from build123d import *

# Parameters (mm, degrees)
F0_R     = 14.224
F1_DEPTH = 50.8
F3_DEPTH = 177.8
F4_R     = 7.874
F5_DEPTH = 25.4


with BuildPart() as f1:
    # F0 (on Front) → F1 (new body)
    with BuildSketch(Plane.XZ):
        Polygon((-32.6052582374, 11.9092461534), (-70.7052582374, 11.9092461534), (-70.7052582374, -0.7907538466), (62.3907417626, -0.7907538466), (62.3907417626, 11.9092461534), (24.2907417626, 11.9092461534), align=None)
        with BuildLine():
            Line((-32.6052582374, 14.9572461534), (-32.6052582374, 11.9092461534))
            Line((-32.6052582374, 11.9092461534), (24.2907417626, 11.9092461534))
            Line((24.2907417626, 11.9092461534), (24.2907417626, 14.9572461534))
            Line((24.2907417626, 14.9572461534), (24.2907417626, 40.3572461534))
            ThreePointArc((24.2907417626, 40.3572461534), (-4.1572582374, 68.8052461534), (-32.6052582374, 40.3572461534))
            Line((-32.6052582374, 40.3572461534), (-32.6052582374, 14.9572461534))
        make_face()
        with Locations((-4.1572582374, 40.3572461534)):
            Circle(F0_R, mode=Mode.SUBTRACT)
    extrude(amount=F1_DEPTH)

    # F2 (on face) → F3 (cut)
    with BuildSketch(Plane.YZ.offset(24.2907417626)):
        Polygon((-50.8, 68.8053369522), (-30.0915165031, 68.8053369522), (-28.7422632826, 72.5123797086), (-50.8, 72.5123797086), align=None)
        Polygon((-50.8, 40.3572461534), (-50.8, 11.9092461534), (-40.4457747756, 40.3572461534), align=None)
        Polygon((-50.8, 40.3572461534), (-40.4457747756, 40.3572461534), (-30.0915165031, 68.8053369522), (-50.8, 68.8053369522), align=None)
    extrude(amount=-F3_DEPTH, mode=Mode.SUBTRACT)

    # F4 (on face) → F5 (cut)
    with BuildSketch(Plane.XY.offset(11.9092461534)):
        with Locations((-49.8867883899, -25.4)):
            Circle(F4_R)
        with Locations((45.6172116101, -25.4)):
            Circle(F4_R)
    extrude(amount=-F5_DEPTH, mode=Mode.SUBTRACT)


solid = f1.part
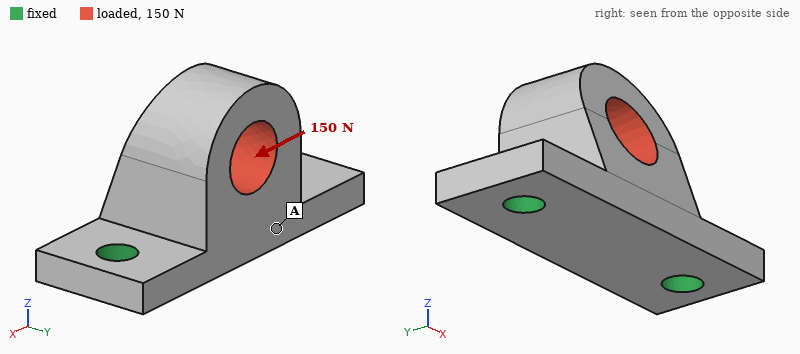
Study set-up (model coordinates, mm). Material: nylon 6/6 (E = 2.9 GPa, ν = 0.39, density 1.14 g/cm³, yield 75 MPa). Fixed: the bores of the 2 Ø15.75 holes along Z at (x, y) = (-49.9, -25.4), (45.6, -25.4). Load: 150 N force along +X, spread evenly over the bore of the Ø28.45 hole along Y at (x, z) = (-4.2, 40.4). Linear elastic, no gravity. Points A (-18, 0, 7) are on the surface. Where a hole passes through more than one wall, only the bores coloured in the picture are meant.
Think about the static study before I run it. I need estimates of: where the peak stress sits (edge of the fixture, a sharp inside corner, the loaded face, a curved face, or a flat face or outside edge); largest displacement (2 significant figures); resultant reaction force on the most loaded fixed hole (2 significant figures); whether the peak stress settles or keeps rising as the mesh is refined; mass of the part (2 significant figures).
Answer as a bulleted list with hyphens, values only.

- edge of the fixture
- 16 µm
- 100 N
- keeps rising
- 200 g
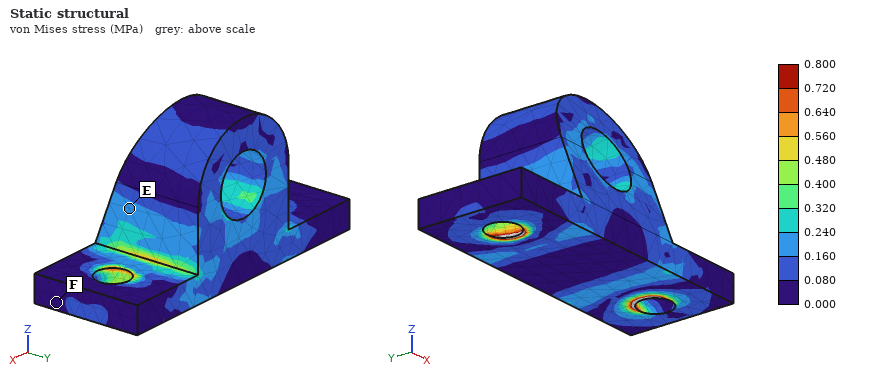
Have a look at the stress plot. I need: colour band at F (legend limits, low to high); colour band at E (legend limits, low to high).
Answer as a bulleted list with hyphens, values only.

- 0.000 to 0.080 MPa
- 0.160 to 0.240 MPa
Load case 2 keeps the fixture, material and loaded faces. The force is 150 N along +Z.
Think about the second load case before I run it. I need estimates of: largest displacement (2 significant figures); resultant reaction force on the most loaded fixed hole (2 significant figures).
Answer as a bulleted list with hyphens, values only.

- 16 µm
- 85 N
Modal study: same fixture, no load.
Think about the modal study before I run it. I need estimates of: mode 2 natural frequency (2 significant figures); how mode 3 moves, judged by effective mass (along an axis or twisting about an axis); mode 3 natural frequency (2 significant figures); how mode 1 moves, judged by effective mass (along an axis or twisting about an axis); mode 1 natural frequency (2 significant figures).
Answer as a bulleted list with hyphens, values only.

- 1800 Hz
- along Z
- 2000 Hz
- along Y
- 840 Hz
